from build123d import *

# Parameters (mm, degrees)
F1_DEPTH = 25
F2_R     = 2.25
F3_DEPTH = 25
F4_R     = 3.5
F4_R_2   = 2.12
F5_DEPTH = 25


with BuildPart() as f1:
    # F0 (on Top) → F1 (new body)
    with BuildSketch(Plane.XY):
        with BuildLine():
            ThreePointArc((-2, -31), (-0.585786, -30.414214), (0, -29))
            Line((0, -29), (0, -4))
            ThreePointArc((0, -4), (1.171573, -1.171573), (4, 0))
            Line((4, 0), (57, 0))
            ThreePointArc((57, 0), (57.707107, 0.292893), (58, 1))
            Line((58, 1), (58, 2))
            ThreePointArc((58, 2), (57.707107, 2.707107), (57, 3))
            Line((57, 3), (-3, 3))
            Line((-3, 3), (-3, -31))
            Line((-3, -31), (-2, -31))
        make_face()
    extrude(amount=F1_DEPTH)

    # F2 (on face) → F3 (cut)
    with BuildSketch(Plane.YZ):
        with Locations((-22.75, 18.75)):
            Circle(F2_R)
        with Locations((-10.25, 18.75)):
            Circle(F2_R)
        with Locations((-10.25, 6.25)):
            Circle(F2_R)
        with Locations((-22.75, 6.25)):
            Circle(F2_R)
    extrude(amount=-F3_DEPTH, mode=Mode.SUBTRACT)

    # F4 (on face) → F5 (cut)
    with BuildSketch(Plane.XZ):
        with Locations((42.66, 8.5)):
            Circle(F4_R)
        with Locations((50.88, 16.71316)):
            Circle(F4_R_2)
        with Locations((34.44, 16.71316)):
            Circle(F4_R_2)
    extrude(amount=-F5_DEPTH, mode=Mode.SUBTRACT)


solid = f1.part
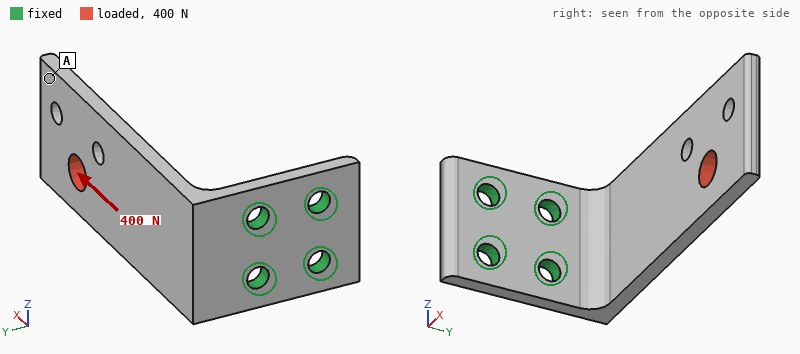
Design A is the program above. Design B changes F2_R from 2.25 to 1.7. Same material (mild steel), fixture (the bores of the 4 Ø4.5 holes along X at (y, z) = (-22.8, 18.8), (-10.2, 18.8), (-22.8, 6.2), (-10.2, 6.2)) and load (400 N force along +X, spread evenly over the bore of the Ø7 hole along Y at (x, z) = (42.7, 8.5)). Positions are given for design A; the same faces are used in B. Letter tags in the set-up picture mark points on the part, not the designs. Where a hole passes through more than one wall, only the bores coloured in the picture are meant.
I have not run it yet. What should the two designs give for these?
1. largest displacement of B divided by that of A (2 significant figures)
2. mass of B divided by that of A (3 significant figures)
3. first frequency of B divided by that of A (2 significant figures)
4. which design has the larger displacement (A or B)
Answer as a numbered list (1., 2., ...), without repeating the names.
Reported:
1. 1.1
2. 1.01
3. 0.98
4. B
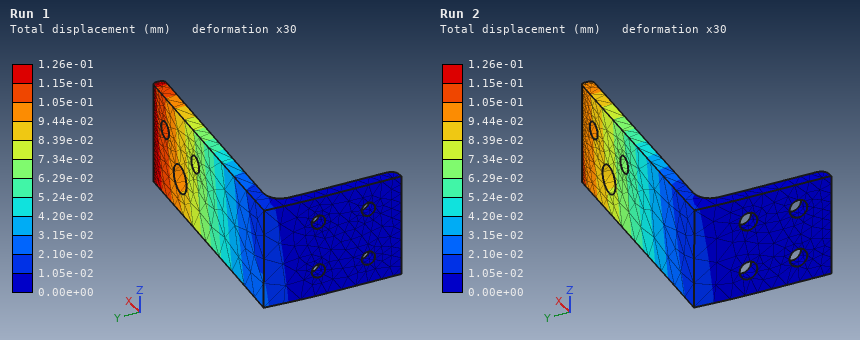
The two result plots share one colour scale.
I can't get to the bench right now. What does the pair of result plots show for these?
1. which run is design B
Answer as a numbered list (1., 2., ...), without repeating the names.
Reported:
1. Run 1
